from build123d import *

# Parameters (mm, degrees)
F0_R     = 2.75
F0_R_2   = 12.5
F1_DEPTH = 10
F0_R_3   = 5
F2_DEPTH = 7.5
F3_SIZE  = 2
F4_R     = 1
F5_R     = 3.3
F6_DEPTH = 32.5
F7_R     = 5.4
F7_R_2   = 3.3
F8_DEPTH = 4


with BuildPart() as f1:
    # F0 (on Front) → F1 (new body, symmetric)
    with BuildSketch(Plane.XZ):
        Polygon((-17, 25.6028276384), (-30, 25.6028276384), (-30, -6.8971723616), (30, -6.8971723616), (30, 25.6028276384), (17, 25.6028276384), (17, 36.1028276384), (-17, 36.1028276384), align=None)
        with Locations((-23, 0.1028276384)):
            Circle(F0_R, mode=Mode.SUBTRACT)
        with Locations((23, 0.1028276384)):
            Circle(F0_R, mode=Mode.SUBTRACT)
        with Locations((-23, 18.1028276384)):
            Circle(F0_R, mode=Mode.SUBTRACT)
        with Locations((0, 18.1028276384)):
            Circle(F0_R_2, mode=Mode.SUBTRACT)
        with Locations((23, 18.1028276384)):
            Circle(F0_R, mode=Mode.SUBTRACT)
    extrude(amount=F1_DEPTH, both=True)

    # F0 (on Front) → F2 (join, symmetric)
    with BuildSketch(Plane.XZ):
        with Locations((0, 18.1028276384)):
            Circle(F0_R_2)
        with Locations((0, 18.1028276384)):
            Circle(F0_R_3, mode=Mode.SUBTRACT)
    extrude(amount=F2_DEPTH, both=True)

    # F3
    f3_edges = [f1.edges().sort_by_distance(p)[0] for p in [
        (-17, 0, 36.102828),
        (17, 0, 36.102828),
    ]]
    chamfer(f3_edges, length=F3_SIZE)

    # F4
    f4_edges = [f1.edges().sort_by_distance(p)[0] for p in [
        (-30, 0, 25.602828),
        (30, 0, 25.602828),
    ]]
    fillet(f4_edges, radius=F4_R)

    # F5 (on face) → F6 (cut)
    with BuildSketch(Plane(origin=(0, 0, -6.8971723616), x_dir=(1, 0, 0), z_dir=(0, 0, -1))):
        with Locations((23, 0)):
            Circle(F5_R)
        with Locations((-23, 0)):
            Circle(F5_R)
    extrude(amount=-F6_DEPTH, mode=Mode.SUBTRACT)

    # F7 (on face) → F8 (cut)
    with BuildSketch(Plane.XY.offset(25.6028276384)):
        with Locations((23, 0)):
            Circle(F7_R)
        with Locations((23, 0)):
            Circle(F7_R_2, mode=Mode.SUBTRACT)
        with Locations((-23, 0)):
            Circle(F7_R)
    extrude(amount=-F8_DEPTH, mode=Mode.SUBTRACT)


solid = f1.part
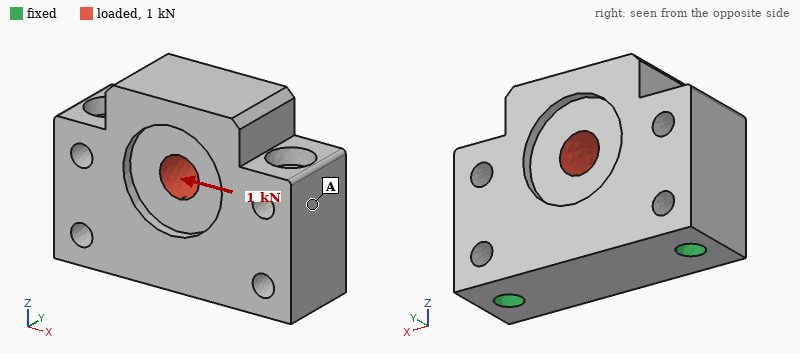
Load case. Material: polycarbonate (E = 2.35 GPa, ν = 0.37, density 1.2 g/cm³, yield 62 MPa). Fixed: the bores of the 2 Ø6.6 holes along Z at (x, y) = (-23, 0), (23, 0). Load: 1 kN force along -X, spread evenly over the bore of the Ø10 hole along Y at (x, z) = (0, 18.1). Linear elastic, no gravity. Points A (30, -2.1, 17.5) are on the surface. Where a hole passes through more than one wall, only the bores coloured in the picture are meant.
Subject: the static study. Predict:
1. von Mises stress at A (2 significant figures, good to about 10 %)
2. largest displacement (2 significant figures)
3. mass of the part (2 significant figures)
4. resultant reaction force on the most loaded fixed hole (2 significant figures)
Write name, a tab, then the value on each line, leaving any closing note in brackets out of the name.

von Mises stress at A	0.93 MPa
largest displacement	21 µm
mass of the part	46 g
resultant reaction force on the most loaded fixed hole	520 N
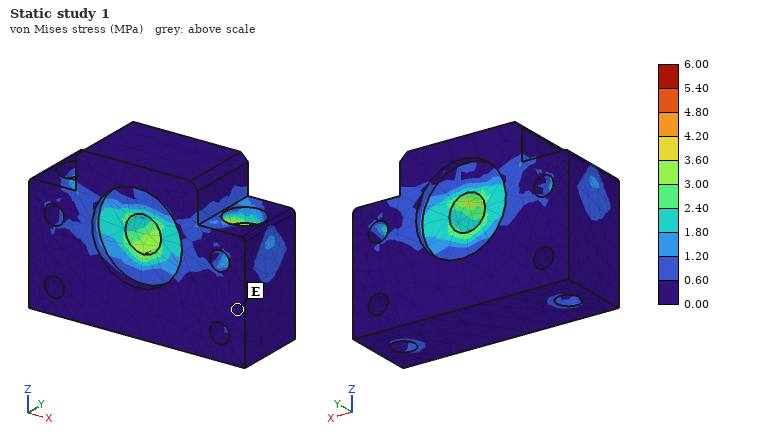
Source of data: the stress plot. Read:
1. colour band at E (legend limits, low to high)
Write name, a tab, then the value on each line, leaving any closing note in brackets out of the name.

colour band at E	0.00 to 0.60 MPa
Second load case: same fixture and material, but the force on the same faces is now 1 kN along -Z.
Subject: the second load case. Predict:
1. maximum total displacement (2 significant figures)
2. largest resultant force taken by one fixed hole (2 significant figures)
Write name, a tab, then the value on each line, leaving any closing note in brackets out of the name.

maximum total displacement	29 µm
largest resultant force taken by one fixed hole	520 N
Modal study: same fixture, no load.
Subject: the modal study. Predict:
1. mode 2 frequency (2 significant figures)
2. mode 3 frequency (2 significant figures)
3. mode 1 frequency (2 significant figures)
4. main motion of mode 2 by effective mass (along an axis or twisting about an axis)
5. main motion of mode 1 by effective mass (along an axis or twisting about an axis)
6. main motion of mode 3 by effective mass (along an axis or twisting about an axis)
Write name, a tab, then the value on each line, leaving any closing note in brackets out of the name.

mode 2 frequency	6700 Hz
mode 3 frequency	7600 Hz
mode 1 frequency	3800 Hz
main motion of mode 2 by effective mass	along Y
main motion of mode 1 by effective mass	along Y
main motion of mode 3 by effective mass	along Z
